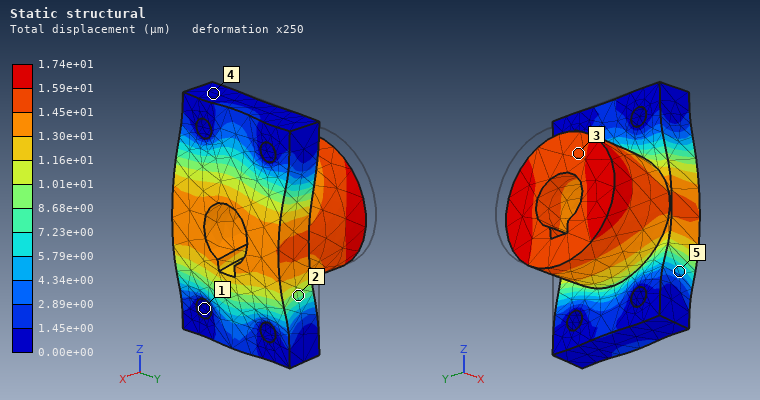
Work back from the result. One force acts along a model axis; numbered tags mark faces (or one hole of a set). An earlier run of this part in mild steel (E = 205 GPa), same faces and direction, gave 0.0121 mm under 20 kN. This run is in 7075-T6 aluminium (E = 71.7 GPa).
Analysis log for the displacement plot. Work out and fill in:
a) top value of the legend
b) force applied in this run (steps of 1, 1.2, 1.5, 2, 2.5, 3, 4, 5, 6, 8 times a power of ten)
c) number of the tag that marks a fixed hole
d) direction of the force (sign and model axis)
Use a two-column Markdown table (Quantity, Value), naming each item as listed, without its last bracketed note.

| Quantity | Value |
|---|---|
| top value of the legend | 1.74e+01 µm |
| force applied in this run | 10 kN |
| number of the tag that marks a fixed hole | 1 |
| direction of the force | +X |
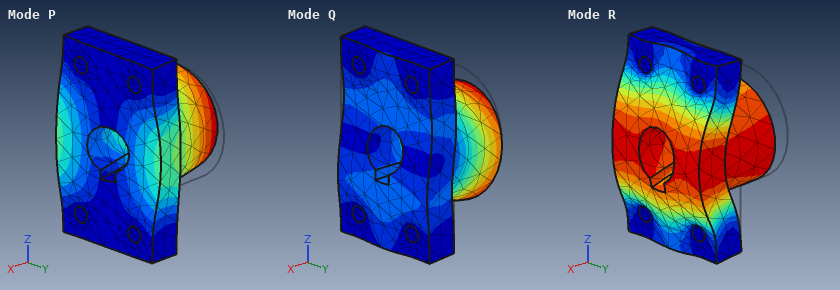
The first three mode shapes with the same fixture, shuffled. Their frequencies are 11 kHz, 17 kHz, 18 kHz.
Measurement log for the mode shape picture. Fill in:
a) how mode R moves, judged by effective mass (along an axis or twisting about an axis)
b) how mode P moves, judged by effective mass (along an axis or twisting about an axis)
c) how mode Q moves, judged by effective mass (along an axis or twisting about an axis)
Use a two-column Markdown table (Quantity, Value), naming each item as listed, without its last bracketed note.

| Quantity | Value |
|---|---|
| how mode R moves, judged by effective mass | along X |
| how mode P moves, judged by effective mass | along Y |
| how mode Q moves, judged by effective mass | along Z |
